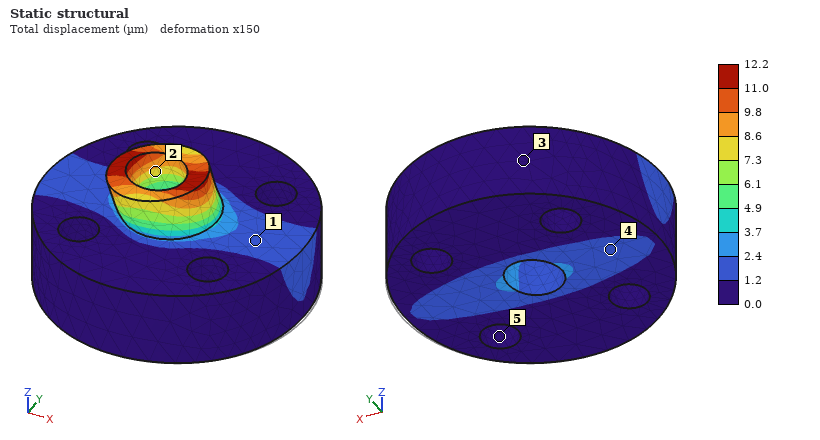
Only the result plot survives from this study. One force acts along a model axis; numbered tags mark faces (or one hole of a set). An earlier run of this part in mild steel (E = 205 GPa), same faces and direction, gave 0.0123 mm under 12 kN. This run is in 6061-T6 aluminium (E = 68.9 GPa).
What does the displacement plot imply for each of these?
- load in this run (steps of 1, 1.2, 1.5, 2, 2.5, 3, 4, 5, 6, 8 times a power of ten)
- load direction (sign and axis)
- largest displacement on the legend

4 kN
-X
12.2 µm
